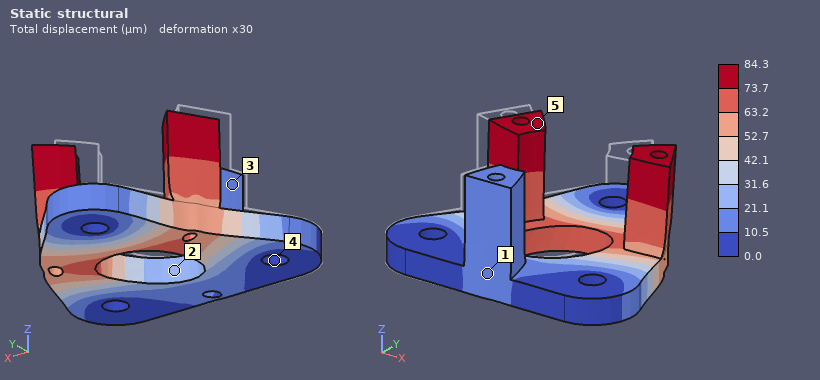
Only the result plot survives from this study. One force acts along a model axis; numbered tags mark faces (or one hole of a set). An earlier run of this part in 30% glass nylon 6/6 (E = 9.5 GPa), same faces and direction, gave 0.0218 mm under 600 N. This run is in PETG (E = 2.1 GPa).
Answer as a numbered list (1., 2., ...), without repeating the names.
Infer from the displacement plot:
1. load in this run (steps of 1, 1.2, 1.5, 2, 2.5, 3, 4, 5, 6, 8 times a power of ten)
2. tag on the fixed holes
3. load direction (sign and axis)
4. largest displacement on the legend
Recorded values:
1. 500 N
2. 4
3. +X
4. 84.3 µm
